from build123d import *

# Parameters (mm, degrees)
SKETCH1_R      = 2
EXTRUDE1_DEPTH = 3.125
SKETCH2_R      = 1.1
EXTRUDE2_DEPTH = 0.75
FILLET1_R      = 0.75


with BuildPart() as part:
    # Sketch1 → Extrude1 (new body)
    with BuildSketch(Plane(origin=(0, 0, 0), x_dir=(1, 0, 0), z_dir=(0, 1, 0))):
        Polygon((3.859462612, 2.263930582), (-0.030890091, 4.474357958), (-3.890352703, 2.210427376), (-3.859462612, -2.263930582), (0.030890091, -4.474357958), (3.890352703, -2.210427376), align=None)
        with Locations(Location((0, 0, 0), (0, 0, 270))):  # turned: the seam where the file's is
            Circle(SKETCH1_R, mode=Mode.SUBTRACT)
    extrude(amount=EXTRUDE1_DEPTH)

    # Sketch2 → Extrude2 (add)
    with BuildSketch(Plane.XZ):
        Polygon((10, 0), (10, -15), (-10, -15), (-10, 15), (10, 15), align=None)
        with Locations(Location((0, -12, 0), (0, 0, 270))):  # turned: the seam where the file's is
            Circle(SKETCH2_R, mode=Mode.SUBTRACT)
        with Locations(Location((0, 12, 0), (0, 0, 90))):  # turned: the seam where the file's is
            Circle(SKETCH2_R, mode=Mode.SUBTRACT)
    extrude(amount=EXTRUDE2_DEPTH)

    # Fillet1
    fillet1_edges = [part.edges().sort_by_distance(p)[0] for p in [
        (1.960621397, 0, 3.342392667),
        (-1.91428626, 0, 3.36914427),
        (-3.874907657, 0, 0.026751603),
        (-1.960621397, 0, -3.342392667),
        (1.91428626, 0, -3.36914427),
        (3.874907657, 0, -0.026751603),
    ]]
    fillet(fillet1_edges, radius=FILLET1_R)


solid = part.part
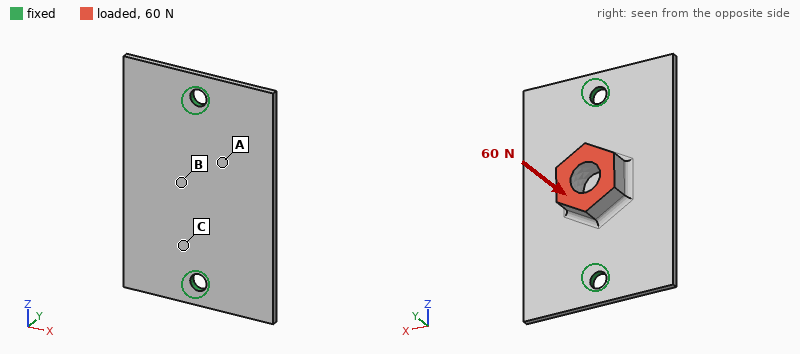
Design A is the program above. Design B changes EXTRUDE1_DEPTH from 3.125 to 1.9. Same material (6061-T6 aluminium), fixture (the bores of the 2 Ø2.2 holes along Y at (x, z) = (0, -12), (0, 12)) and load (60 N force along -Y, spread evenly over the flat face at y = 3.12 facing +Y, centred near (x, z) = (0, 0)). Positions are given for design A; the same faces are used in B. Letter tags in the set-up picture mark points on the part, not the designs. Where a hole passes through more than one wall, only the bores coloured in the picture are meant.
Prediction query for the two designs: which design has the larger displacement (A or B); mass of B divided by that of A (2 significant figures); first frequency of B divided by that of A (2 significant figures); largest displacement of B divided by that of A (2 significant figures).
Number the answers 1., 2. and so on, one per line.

1. B
2. 0.92
3. 1.0
4. 1.1
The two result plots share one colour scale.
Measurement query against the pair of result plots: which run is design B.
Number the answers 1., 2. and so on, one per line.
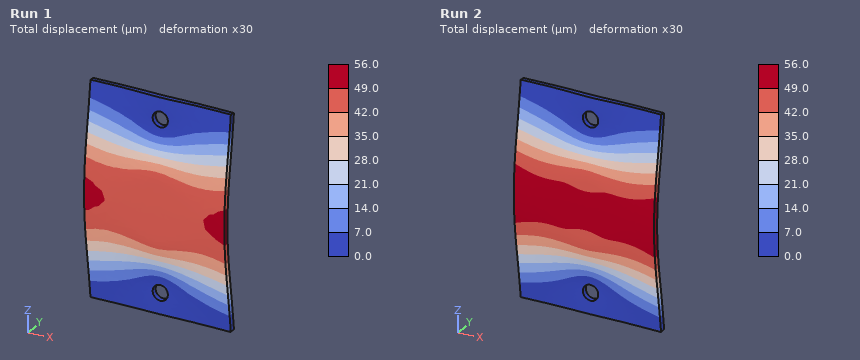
1. Run 2
